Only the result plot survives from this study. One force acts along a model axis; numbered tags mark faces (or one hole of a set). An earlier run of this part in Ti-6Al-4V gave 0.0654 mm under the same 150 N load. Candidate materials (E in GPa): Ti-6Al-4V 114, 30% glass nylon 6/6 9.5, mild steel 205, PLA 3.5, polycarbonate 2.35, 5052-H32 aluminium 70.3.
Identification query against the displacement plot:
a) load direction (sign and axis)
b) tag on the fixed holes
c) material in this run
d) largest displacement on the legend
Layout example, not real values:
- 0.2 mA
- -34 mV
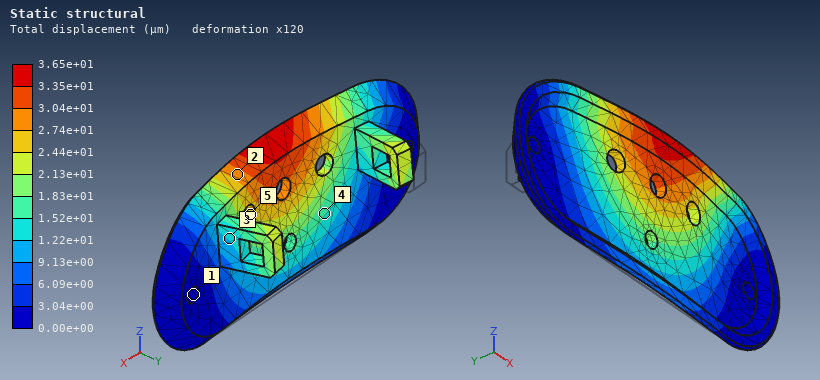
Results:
- -Y
- 1
- mild steel
- 3.65e+01 µm
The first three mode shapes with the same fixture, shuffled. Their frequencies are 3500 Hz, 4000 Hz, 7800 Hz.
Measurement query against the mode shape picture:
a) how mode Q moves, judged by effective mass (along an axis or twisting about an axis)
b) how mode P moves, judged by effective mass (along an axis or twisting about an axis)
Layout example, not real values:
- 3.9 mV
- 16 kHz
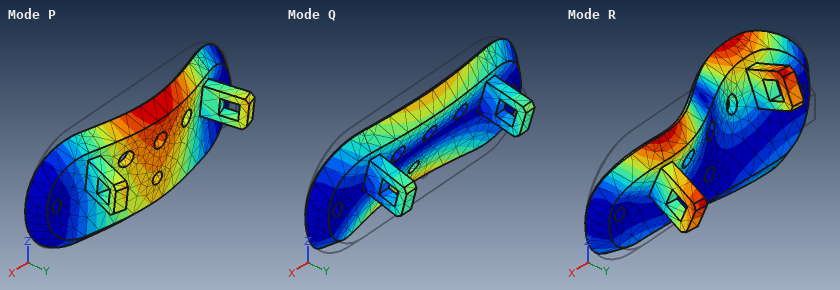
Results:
- twisting about X
- along Y
